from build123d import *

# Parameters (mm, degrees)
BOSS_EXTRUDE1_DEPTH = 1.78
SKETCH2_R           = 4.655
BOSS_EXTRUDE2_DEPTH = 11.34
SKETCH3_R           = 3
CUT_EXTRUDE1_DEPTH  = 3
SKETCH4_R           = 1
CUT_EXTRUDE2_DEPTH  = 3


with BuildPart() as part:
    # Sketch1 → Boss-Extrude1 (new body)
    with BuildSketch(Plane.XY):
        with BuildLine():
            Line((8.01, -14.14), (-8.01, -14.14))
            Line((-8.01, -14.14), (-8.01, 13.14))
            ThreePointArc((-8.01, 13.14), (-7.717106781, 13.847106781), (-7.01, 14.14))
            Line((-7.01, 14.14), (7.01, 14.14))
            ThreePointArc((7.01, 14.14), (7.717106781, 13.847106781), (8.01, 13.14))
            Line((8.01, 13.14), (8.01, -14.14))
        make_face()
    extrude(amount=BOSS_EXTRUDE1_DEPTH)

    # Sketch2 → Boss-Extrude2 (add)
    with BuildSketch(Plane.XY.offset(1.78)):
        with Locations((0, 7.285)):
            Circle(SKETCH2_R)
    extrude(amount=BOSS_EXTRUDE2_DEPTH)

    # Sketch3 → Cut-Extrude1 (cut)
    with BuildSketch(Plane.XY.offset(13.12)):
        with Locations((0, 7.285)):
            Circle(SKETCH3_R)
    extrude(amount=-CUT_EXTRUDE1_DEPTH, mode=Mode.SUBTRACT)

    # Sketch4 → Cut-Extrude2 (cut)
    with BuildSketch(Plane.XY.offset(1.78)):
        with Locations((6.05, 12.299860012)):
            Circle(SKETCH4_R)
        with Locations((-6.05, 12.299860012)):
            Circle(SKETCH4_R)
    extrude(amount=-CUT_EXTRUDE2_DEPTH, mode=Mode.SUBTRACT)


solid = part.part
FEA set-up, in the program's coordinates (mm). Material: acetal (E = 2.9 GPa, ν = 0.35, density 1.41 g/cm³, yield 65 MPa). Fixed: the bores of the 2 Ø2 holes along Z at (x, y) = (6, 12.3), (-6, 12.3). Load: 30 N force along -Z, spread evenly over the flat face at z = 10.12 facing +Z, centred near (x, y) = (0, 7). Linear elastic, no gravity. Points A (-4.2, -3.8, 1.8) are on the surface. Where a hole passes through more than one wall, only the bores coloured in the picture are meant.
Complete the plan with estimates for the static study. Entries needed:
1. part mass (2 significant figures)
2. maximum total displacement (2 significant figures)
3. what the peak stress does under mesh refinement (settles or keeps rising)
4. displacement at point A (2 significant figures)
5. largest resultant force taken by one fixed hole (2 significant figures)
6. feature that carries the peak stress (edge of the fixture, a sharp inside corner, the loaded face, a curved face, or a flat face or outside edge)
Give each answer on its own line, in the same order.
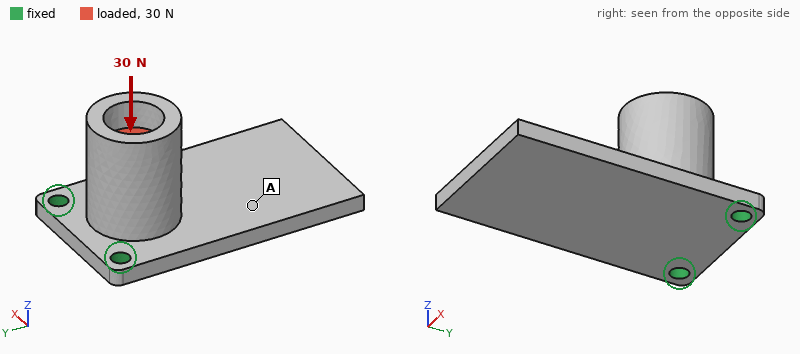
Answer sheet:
2.1 g
0.40 mm
keeps rising
0.23 mm
15 N
edge of the fixture
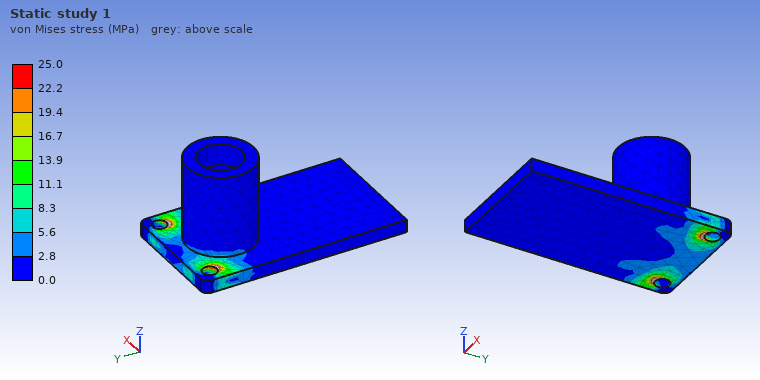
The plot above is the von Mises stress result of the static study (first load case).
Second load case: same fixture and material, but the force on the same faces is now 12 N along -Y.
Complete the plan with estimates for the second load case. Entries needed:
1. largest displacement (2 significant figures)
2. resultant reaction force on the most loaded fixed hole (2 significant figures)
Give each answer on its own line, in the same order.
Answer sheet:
0.39 mm
6.5 N
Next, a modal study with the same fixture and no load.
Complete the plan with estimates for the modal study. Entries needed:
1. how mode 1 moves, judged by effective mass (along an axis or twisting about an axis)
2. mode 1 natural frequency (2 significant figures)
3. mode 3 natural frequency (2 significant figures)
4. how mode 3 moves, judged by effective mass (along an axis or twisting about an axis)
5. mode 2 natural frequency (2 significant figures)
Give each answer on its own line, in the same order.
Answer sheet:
along Z
700 Hz
2600 Hz
twisting about Y
2500 Hz
